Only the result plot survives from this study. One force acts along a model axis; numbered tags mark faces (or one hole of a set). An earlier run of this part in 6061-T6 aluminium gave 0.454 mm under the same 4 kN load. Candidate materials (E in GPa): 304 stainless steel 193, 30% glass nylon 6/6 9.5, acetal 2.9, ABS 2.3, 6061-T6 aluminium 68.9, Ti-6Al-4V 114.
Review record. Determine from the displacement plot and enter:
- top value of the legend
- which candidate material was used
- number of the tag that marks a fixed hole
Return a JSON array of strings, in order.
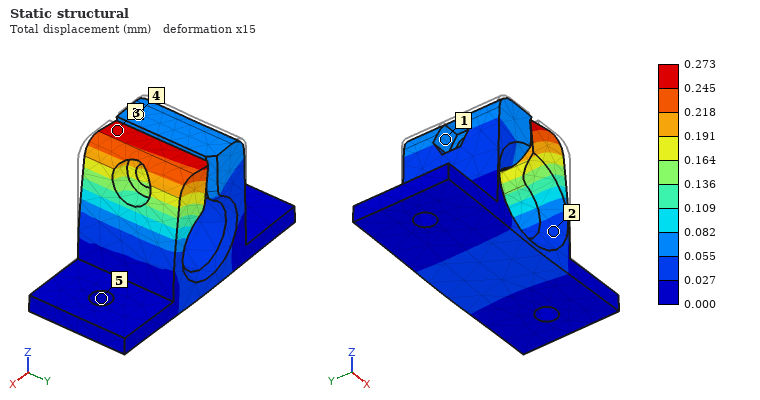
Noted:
["0.273 mm", "Ti-6Al-4V", "5"]
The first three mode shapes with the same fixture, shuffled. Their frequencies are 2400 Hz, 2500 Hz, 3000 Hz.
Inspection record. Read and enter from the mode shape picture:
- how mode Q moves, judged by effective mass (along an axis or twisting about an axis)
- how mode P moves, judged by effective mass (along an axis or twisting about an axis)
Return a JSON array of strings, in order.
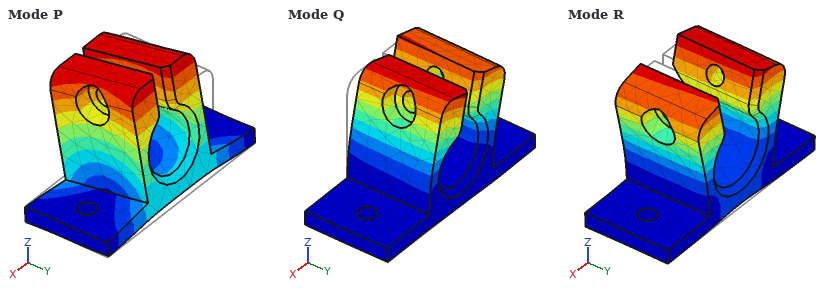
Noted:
["along X", "along Y"]
